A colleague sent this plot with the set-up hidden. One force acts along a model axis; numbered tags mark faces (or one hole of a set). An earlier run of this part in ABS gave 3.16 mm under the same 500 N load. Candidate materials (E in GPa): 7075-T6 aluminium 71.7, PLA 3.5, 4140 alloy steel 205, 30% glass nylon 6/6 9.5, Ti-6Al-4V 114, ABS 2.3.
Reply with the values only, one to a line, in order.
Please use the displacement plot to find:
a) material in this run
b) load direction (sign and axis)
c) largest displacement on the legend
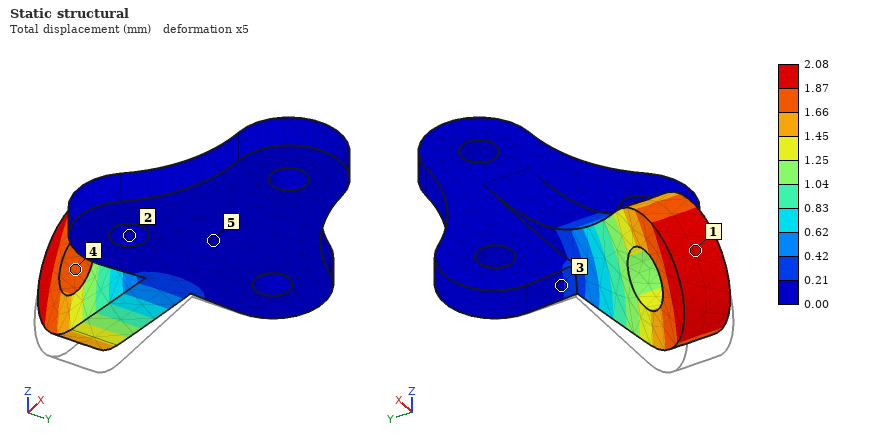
PLA
+Z
2.08 mm
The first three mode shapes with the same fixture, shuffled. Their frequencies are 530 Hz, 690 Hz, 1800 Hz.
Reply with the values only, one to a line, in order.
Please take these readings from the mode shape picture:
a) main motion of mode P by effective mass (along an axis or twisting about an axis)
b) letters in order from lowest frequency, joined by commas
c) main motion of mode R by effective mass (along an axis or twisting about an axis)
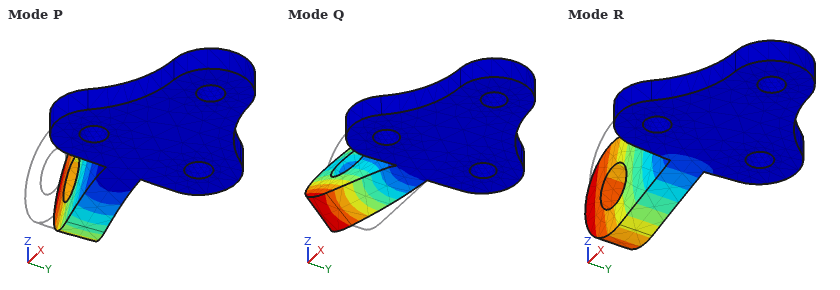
along Y
R, P, Q
along Z
